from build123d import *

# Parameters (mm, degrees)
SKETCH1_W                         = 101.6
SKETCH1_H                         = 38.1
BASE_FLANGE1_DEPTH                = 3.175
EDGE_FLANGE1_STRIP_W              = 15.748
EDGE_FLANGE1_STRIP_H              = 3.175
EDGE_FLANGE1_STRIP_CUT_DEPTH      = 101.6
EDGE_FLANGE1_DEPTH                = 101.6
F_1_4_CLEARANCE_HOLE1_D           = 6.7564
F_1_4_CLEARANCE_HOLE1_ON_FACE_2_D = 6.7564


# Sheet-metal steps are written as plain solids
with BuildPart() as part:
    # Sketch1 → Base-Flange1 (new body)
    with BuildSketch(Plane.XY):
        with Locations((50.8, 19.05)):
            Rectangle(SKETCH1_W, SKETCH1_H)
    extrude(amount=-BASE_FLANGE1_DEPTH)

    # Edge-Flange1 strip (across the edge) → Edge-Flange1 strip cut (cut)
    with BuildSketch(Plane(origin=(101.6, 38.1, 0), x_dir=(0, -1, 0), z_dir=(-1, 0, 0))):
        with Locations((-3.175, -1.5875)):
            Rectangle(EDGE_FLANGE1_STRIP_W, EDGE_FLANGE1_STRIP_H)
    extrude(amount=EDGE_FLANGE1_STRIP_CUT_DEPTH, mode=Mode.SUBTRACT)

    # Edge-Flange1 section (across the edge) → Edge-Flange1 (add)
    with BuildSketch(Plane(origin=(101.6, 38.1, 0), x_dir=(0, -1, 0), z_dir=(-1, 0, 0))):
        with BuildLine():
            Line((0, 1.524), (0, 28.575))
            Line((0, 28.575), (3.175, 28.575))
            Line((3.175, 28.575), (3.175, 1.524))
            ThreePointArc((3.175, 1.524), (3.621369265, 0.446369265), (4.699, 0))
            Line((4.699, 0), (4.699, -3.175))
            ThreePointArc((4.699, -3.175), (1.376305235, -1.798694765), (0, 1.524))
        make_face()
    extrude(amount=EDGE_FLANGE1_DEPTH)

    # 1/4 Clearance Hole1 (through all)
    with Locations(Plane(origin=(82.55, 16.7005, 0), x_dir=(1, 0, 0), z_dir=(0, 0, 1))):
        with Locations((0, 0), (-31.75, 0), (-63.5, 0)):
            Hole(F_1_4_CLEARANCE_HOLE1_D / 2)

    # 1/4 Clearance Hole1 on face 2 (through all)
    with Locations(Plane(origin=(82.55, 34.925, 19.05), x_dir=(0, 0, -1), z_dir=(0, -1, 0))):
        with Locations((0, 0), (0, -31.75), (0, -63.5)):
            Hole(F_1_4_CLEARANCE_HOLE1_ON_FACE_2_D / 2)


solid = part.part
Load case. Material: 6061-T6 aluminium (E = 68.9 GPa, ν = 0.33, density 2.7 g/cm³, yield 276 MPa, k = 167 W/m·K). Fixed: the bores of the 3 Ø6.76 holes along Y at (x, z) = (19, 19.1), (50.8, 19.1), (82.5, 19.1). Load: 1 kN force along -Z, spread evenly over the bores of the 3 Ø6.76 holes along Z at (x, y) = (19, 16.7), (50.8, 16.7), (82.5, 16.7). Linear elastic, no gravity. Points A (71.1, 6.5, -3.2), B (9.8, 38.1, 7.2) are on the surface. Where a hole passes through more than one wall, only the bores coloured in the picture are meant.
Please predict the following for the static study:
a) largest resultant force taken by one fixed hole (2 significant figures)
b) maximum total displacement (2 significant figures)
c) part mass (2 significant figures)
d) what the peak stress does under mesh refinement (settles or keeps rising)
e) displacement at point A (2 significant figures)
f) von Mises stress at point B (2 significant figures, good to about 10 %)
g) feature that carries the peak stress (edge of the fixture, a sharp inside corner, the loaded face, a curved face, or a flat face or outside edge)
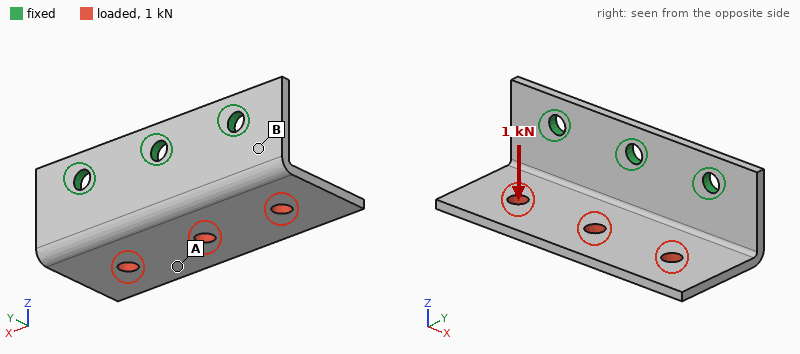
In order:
360 N
1.0 mm
55 g
keeps rising
0.82 mm
94 MPa
edge of the fixture
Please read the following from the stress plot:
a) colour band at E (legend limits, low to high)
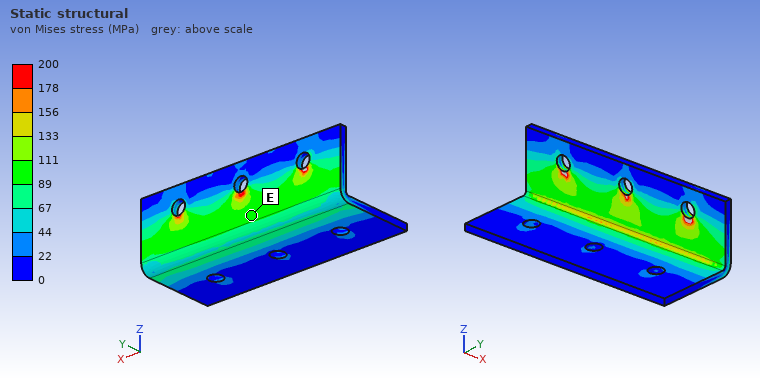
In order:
89 to 111 MPa
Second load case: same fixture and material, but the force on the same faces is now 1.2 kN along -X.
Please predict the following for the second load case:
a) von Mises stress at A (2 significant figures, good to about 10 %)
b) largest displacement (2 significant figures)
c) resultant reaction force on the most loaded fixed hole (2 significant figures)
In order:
12 MPa
0.24 mm
600 N
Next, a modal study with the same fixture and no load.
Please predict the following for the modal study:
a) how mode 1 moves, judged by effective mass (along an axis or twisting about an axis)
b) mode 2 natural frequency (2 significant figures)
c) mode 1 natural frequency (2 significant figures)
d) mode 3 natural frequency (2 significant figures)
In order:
along Z
1600 Hz
1100 Hz
3100 Hz
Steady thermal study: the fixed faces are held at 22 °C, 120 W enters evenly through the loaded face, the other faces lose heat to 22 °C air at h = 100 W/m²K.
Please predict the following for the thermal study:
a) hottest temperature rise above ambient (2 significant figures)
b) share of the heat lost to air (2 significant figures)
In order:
74 K
40 %
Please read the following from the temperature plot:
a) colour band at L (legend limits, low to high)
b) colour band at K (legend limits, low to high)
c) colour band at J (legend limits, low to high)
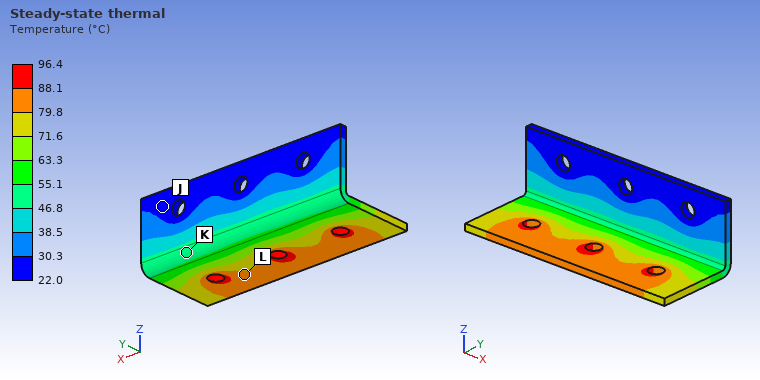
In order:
79.8 to 88.1 °C
46.8 to 55.1 °C
22.0 to 30.3 °C
